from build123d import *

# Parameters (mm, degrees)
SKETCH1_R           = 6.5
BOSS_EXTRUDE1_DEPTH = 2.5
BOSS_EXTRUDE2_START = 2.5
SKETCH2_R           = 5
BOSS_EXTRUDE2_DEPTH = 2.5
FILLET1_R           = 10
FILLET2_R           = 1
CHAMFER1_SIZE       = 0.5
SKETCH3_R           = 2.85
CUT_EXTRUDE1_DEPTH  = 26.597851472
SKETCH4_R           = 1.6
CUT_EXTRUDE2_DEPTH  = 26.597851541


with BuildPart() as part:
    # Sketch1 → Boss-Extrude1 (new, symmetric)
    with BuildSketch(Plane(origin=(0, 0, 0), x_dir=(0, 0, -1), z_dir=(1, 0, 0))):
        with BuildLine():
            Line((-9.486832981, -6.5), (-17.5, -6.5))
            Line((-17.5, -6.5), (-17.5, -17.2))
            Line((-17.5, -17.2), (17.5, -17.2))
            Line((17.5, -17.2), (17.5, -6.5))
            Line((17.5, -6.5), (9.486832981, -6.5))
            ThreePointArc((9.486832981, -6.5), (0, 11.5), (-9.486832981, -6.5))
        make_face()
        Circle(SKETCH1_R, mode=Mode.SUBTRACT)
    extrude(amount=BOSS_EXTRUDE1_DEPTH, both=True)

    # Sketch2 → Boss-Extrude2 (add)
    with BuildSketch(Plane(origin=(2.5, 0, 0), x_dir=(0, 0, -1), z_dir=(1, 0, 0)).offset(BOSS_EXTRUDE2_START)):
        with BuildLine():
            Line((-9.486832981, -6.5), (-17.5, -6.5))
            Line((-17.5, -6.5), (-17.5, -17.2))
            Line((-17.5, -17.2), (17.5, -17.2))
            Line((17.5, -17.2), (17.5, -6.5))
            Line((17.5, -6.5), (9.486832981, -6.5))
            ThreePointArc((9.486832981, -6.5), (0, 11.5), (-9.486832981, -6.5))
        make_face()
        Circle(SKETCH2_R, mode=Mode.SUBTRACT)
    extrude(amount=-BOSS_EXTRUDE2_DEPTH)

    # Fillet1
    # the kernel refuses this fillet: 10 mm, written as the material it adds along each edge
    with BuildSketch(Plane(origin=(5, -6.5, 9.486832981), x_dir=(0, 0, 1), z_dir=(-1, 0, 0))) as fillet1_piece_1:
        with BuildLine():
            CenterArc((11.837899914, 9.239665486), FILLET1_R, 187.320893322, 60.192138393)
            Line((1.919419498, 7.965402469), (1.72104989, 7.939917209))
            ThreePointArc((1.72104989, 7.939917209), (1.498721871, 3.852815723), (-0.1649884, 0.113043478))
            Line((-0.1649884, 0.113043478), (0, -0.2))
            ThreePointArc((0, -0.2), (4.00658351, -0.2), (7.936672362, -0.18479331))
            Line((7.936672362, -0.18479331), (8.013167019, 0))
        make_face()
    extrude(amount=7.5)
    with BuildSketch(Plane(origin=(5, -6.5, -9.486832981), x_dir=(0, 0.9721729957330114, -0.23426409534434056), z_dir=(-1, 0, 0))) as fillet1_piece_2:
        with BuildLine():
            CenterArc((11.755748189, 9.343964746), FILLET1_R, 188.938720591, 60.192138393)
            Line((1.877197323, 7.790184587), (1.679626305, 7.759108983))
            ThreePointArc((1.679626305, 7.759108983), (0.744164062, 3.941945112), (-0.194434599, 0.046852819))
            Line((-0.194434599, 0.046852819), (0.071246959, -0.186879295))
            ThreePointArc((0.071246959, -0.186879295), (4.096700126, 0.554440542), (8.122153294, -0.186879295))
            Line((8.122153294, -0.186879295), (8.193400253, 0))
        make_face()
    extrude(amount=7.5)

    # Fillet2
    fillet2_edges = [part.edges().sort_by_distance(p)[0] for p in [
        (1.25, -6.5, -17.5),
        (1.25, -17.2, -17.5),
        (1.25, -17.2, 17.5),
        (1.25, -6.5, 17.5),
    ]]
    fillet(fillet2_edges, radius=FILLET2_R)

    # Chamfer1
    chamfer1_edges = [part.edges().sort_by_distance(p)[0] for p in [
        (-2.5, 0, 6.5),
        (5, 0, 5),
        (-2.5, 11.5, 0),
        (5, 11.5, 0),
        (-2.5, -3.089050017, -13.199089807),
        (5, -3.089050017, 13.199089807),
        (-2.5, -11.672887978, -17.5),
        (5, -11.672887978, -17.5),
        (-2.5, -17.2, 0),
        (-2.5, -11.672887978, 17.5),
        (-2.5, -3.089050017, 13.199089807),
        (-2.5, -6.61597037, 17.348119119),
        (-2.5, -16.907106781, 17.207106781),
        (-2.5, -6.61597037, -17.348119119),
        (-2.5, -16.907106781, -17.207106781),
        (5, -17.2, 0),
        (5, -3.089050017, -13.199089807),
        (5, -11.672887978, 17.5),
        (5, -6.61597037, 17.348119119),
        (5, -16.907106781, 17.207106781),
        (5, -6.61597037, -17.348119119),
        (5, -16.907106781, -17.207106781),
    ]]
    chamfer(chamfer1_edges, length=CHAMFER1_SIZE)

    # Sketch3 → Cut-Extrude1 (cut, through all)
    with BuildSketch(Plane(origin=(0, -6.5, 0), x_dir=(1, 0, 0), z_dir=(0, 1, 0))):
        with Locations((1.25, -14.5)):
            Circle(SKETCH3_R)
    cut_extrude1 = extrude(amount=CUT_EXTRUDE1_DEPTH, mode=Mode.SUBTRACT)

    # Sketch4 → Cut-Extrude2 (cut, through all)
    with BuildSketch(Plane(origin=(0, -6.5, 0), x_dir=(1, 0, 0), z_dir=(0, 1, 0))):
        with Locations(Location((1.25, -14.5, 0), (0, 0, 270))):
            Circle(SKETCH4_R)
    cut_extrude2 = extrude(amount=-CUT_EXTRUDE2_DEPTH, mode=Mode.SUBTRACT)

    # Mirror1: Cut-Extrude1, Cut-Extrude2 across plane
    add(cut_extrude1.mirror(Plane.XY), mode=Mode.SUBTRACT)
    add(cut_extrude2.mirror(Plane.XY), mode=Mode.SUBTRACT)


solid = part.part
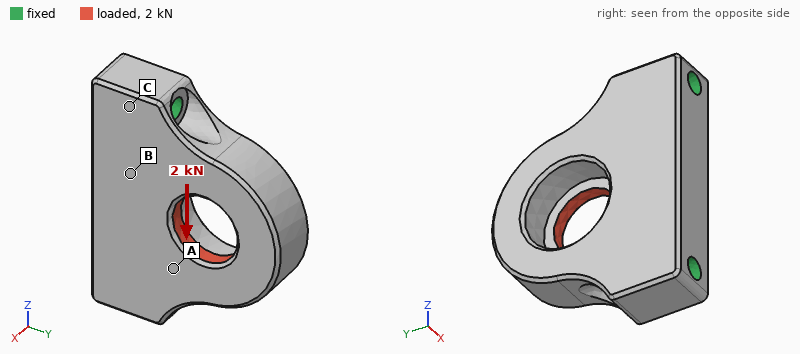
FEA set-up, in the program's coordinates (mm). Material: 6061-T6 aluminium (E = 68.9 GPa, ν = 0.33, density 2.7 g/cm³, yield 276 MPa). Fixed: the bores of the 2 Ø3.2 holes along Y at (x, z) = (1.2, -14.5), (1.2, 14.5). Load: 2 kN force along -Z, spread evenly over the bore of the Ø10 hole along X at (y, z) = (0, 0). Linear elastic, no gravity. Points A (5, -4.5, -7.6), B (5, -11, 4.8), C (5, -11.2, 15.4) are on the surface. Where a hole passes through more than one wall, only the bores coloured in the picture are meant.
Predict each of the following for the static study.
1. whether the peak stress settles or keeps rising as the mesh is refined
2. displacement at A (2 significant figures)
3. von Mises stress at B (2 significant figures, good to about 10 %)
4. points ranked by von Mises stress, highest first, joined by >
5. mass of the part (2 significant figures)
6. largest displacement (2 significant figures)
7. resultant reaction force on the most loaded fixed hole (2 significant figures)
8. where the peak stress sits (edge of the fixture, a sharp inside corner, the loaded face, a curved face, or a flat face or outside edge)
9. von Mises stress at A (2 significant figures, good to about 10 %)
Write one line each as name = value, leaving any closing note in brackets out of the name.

whether the peak stress settles or keeps rising as the mesh is refined = keeps rising
displacement at A = 4.3 µm
von Mises stress at B = 13 MPa
points ranked by von Mises stress, highest first, joined by > = A > B > C
mass of the part = 12 g
largest displacement = 19 µm
resultant reaction force on the most loaded fixed hole = 1.2 kN
where the peak stress sits = a sharp inside corner
von Mises stress at A = 36 MPa
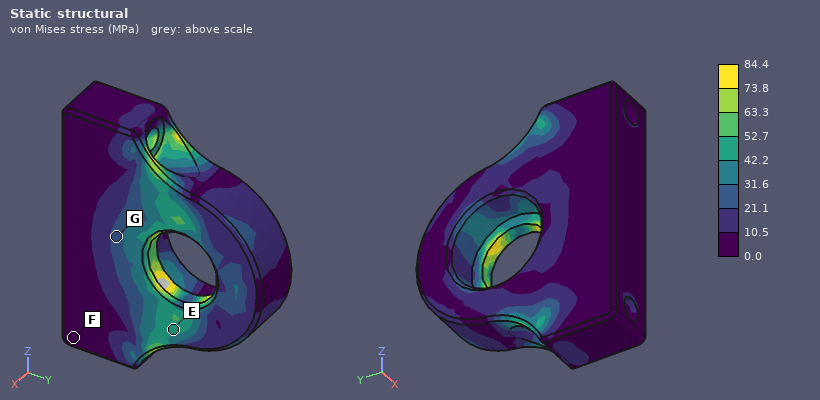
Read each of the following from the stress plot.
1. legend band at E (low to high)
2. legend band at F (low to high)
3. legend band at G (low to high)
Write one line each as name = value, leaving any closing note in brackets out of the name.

legend band at E = 42.2 to 52.7 MPa
legend band at F = 0.0 to 10.5 MPa
legend band at G = 21.1 to 31.6 MPa
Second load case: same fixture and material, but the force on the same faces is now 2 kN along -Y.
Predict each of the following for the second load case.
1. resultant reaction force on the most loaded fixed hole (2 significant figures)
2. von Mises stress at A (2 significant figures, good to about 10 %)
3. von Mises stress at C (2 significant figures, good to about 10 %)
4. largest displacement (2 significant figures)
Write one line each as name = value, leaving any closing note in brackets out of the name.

resultant reaction force on the most loaded fixed hole = 1.1 kN
von Mises stress at A = 27 MPa
von Mises stress at C = 10 MPa
largest displacement = 26 µm
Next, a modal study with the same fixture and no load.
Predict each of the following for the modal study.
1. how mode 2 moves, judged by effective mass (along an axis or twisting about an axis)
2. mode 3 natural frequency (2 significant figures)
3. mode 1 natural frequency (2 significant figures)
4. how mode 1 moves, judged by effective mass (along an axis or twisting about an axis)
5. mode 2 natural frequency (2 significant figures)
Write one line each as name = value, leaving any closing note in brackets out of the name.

how mode 2 moves, judged by effective mass = along Z
mode 3 natural frequency = 27 kHz
mode 1 natural frequency = 11 kHz
how mode 1 moves, judged by effective mass = along X
mode 2 natural frequency = 24 kHz
